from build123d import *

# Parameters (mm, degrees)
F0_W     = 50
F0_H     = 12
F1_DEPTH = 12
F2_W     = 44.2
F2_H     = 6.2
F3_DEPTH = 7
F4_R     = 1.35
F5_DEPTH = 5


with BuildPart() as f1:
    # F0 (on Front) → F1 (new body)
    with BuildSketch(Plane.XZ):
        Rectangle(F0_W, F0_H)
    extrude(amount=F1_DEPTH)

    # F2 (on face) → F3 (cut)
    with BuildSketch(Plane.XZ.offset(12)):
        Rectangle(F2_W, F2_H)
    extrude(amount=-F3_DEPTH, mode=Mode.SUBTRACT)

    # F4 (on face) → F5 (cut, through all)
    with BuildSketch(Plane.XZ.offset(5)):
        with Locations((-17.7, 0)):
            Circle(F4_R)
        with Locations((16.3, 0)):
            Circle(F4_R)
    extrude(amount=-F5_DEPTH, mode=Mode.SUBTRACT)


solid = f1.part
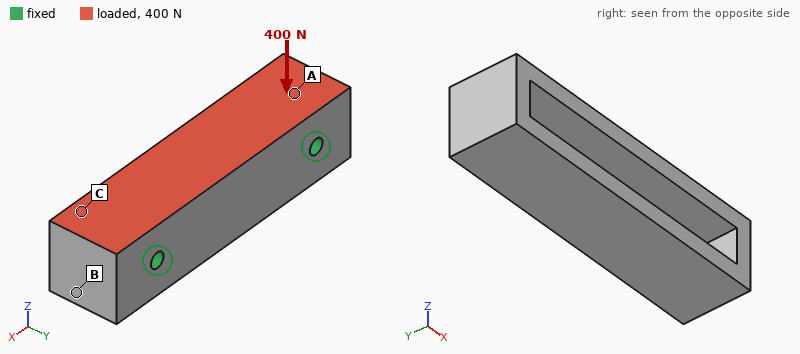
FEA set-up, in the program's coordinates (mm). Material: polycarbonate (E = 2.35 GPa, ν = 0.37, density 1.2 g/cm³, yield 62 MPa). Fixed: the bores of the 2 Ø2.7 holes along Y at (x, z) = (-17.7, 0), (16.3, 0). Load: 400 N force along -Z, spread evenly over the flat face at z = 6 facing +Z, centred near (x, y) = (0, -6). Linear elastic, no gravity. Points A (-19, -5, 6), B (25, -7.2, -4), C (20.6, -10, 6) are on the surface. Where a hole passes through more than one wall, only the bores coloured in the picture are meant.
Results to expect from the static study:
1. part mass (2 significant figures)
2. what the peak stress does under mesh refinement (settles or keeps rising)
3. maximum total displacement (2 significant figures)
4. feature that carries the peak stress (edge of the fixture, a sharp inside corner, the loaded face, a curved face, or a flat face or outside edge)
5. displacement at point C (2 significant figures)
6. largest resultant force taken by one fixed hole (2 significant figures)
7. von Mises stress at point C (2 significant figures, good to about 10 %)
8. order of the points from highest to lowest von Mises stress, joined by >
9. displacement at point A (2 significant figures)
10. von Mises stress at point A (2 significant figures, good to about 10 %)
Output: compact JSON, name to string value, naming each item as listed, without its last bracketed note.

{"part mass": "6.3 g", "what the peak stress does under mesh refinement": "keeps rising", "maximum total displacement": "0.24 mm", "feature that carries the peak stress": "edge of the fixture", "displacement at point C": "0.070 mm", "largest resultant force taken by one fixed hole": "210 N", "von Mises stress at point C": "4.2 MPa", "order of the points from highest to lowest von Mises stress, joined by >": "A > C > B", "displacement at point A": "0.040 mm", "von Mises stress at point A": "7.2 MPa"}
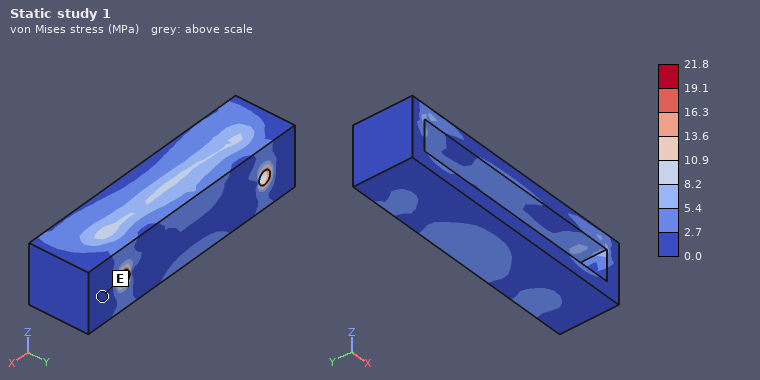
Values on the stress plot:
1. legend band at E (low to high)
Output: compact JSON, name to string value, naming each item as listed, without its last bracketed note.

{"legend band at E": "0.0 to 2.7 MPa"}
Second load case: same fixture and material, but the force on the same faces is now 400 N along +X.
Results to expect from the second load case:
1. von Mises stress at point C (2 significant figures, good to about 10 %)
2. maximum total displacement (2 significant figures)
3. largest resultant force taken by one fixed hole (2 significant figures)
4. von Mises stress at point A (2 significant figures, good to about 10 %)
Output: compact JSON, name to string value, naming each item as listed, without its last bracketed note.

{"von Mises stress at point C": "2.0 MPa", "maximum total displacement": "49 µm", "largest resultant force taken by one fixed hole": "220 N", "von Mises stress at point A": "2.3 MPa"}
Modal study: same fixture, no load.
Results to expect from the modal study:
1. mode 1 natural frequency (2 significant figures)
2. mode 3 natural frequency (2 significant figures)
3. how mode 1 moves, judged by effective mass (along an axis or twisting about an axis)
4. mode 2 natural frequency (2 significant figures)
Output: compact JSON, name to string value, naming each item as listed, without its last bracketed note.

{"mode 1 natural frequency": "4300 Hz", "mode 3 natural frequency": "6300 Hz", "how mode 1 moves, judged by effective mass": "along Z", "mode 2 natural frequency": "6100 Hz"}
